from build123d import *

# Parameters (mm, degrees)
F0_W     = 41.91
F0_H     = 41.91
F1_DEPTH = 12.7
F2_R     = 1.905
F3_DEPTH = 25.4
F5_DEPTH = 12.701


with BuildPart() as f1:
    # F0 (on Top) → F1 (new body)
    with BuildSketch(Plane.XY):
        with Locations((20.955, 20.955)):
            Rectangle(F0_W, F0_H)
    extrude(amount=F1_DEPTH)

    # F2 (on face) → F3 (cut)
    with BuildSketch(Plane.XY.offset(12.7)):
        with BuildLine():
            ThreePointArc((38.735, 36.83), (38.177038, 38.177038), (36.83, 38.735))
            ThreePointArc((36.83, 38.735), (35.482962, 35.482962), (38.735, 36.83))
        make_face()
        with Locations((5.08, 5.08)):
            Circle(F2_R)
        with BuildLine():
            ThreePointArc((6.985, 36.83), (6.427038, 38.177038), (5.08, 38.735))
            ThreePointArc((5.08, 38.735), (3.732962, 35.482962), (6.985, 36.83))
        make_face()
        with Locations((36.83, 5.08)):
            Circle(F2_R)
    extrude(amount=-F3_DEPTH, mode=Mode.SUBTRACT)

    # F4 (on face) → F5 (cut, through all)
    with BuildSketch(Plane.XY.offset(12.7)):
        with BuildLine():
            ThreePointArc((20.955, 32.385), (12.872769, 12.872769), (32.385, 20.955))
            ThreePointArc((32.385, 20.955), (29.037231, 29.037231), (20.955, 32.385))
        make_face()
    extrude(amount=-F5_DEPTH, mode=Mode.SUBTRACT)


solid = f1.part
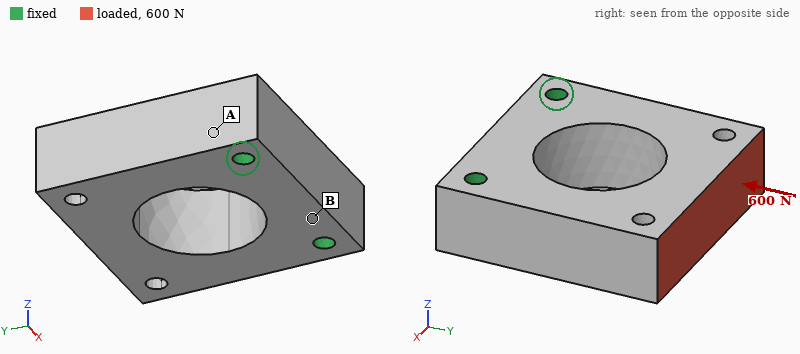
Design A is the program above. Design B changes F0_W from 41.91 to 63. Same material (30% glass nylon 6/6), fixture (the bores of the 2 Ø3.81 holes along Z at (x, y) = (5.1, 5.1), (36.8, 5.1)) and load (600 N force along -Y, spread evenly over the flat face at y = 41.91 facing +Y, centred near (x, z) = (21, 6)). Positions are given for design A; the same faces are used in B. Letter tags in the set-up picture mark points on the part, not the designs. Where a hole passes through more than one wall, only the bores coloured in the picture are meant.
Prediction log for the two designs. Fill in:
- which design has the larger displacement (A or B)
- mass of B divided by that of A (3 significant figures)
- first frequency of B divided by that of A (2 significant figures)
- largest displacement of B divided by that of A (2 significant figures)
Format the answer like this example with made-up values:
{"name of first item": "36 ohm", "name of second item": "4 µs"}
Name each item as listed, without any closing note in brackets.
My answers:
{"which design has the larger displacement": "A", "mass of B divided by that of A": "1.68", "first frequency of B divided by that of A": "0.95", "largest displacement of B divided by that of A": "0.68"}
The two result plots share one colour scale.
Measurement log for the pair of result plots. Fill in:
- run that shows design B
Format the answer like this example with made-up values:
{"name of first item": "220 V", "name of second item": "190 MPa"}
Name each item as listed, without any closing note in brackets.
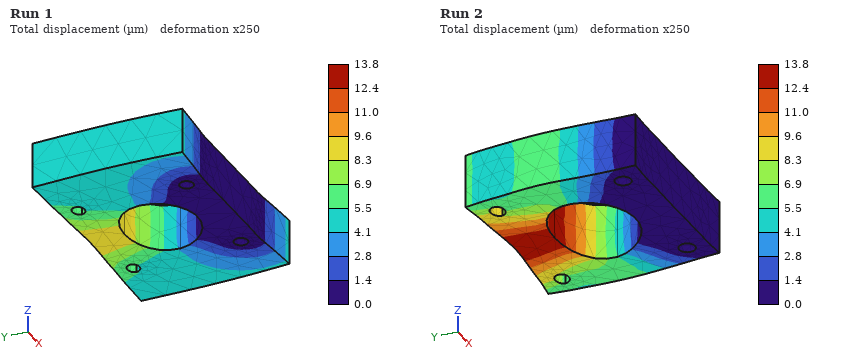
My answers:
{"run that shows design B": "Run 1"}
